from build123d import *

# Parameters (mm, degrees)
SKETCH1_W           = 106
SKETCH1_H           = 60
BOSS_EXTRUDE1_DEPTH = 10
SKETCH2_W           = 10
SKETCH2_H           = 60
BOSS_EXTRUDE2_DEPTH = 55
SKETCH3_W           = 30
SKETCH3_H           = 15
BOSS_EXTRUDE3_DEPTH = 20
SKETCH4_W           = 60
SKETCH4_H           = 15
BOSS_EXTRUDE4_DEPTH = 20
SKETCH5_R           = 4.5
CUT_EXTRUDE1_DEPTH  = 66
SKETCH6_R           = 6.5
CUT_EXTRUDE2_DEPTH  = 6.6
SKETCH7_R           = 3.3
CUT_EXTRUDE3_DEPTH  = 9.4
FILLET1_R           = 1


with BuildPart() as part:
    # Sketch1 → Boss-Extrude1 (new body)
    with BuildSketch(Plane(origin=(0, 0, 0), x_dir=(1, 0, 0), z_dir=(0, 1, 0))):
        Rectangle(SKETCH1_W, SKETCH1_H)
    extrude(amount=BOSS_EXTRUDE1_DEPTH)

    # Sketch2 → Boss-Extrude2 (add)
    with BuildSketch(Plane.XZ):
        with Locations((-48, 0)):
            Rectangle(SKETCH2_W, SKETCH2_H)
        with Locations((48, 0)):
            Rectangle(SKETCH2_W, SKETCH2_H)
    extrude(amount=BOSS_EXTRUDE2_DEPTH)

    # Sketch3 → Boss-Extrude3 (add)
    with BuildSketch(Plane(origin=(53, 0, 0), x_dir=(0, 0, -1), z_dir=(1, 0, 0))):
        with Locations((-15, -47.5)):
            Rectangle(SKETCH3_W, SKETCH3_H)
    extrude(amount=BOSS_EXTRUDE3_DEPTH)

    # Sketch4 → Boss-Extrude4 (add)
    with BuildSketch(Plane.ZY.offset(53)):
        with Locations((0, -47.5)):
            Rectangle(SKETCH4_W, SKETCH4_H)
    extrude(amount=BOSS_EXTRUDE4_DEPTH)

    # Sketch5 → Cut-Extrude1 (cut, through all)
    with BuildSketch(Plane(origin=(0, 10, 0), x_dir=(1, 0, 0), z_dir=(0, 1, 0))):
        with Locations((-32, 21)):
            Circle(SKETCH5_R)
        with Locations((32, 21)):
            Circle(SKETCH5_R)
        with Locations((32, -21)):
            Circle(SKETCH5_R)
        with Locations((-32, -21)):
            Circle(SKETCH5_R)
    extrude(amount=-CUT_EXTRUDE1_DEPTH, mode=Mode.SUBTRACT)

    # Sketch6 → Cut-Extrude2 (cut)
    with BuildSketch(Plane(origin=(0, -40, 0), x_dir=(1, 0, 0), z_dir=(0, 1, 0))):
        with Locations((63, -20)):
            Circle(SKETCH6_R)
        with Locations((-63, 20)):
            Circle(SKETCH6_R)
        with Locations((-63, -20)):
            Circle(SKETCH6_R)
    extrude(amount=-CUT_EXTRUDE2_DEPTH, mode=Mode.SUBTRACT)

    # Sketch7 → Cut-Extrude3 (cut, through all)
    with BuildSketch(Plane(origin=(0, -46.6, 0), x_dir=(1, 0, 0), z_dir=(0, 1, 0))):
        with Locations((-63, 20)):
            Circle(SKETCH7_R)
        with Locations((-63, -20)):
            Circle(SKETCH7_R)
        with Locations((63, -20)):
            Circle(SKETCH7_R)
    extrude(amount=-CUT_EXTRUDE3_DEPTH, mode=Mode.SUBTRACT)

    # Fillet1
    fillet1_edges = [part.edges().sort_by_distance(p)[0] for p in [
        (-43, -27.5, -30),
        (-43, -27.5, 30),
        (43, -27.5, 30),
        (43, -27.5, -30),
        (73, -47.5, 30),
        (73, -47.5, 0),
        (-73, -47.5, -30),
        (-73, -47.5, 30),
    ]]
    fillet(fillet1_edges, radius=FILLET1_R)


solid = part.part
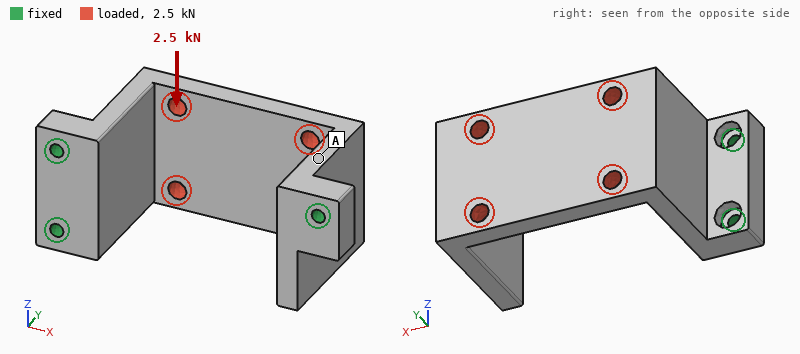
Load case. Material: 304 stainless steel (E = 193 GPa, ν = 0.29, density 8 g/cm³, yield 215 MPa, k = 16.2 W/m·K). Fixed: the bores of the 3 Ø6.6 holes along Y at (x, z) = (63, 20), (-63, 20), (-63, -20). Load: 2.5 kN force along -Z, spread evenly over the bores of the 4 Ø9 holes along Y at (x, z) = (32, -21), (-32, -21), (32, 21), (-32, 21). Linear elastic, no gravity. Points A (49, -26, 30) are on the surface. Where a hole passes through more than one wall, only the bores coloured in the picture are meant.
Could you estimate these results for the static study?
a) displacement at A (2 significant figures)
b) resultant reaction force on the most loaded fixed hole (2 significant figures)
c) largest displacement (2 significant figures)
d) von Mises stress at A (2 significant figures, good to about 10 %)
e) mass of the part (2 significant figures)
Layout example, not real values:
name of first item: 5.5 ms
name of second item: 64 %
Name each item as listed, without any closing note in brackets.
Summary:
displacement at A: 22 µm
resultant reaction force on the most loaded fixed hole: 2.7 kN
largest displacement: 64 µm
von Mises stress at A: 9.4 MPa
mass of the part: 1.2 kg
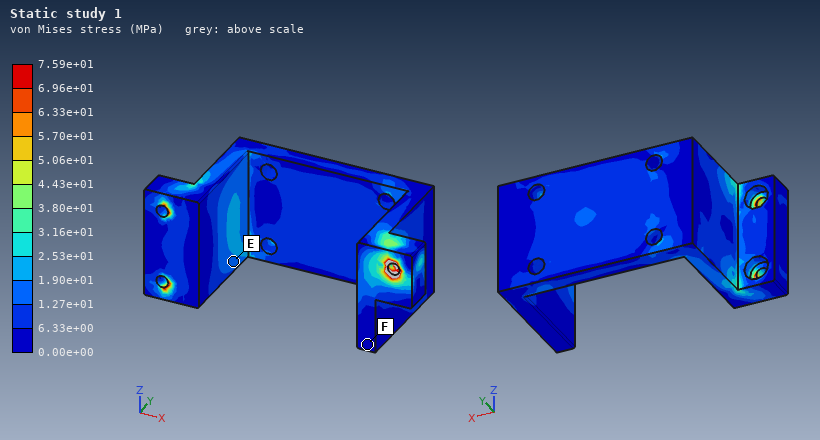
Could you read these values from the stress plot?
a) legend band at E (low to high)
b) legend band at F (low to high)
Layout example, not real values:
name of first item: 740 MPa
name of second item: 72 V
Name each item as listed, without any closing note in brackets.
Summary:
legend band at E: 1.27e+01 to 1.90e+01 MPa
legend band at F: 0.00e+00 to 6.33e+00 MPa
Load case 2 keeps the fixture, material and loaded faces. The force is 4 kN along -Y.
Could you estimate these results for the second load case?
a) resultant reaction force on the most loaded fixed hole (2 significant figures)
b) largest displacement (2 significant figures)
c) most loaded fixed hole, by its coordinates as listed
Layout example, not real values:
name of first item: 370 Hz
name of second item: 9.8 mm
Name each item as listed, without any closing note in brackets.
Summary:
resultant reaction force on the most loaded fixed hole: 2.1 kN
largest displacement: 32 µm
most loaded fixed hole, by its coordinates as listed: (63, 20)
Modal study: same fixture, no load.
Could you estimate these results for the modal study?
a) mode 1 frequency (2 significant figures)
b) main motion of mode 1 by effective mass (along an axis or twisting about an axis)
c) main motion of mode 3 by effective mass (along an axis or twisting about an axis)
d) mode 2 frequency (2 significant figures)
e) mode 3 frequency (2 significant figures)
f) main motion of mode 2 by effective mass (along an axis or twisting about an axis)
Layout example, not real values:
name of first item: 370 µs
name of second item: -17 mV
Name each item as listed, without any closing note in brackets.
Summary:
mode 1 frequency: 1400 Hz
main motion of mode 1 by effective mass: along Z
main motion of mode 3 by effective mass: along Z
mode 2 frequency: 1600 Hz
mode 3 frequency: 3500 Hz
main motion of mode 2 by effective mass: along X
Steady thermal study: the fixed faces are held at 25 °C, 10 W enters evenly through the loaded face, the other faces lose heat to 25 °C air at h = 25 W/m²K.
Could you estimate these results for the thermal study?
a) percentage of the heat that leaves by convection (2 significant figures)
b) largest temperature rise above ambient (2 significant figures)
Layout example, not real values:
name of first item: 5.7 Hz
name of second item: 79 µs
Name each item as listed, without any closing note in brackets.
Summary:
percentage of the heat that leaves by convection: 76 %
largest temperature rise above ambient: 19 K
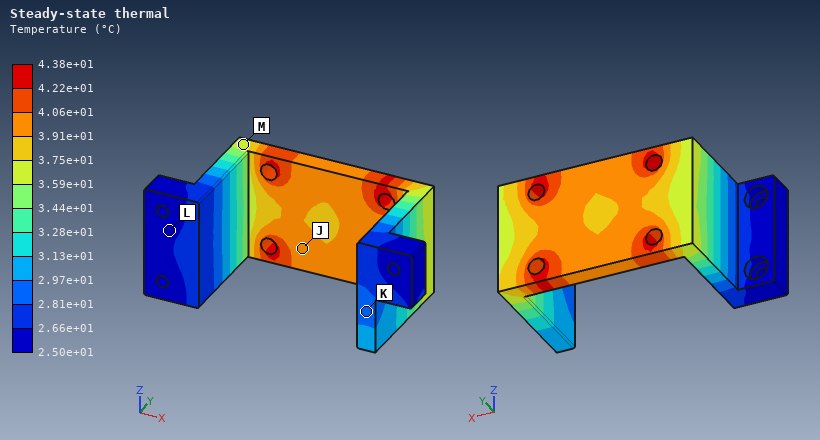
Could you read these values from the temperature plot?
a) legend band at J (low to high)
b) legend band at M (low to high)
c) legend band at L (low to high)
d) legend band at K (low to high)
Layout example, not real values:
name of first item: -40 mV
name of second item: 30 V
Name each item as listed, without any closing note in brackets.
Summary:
legend band at J: 3.91e+01 to 4.06e+01 °C
legend band at M: 3.59e+01 to 3.75e+01 °C
legend band at L: 2.50e+01 to 2.66e+01 °C
legend band at K: 2.81e+01 to 2.97e+01 °C
